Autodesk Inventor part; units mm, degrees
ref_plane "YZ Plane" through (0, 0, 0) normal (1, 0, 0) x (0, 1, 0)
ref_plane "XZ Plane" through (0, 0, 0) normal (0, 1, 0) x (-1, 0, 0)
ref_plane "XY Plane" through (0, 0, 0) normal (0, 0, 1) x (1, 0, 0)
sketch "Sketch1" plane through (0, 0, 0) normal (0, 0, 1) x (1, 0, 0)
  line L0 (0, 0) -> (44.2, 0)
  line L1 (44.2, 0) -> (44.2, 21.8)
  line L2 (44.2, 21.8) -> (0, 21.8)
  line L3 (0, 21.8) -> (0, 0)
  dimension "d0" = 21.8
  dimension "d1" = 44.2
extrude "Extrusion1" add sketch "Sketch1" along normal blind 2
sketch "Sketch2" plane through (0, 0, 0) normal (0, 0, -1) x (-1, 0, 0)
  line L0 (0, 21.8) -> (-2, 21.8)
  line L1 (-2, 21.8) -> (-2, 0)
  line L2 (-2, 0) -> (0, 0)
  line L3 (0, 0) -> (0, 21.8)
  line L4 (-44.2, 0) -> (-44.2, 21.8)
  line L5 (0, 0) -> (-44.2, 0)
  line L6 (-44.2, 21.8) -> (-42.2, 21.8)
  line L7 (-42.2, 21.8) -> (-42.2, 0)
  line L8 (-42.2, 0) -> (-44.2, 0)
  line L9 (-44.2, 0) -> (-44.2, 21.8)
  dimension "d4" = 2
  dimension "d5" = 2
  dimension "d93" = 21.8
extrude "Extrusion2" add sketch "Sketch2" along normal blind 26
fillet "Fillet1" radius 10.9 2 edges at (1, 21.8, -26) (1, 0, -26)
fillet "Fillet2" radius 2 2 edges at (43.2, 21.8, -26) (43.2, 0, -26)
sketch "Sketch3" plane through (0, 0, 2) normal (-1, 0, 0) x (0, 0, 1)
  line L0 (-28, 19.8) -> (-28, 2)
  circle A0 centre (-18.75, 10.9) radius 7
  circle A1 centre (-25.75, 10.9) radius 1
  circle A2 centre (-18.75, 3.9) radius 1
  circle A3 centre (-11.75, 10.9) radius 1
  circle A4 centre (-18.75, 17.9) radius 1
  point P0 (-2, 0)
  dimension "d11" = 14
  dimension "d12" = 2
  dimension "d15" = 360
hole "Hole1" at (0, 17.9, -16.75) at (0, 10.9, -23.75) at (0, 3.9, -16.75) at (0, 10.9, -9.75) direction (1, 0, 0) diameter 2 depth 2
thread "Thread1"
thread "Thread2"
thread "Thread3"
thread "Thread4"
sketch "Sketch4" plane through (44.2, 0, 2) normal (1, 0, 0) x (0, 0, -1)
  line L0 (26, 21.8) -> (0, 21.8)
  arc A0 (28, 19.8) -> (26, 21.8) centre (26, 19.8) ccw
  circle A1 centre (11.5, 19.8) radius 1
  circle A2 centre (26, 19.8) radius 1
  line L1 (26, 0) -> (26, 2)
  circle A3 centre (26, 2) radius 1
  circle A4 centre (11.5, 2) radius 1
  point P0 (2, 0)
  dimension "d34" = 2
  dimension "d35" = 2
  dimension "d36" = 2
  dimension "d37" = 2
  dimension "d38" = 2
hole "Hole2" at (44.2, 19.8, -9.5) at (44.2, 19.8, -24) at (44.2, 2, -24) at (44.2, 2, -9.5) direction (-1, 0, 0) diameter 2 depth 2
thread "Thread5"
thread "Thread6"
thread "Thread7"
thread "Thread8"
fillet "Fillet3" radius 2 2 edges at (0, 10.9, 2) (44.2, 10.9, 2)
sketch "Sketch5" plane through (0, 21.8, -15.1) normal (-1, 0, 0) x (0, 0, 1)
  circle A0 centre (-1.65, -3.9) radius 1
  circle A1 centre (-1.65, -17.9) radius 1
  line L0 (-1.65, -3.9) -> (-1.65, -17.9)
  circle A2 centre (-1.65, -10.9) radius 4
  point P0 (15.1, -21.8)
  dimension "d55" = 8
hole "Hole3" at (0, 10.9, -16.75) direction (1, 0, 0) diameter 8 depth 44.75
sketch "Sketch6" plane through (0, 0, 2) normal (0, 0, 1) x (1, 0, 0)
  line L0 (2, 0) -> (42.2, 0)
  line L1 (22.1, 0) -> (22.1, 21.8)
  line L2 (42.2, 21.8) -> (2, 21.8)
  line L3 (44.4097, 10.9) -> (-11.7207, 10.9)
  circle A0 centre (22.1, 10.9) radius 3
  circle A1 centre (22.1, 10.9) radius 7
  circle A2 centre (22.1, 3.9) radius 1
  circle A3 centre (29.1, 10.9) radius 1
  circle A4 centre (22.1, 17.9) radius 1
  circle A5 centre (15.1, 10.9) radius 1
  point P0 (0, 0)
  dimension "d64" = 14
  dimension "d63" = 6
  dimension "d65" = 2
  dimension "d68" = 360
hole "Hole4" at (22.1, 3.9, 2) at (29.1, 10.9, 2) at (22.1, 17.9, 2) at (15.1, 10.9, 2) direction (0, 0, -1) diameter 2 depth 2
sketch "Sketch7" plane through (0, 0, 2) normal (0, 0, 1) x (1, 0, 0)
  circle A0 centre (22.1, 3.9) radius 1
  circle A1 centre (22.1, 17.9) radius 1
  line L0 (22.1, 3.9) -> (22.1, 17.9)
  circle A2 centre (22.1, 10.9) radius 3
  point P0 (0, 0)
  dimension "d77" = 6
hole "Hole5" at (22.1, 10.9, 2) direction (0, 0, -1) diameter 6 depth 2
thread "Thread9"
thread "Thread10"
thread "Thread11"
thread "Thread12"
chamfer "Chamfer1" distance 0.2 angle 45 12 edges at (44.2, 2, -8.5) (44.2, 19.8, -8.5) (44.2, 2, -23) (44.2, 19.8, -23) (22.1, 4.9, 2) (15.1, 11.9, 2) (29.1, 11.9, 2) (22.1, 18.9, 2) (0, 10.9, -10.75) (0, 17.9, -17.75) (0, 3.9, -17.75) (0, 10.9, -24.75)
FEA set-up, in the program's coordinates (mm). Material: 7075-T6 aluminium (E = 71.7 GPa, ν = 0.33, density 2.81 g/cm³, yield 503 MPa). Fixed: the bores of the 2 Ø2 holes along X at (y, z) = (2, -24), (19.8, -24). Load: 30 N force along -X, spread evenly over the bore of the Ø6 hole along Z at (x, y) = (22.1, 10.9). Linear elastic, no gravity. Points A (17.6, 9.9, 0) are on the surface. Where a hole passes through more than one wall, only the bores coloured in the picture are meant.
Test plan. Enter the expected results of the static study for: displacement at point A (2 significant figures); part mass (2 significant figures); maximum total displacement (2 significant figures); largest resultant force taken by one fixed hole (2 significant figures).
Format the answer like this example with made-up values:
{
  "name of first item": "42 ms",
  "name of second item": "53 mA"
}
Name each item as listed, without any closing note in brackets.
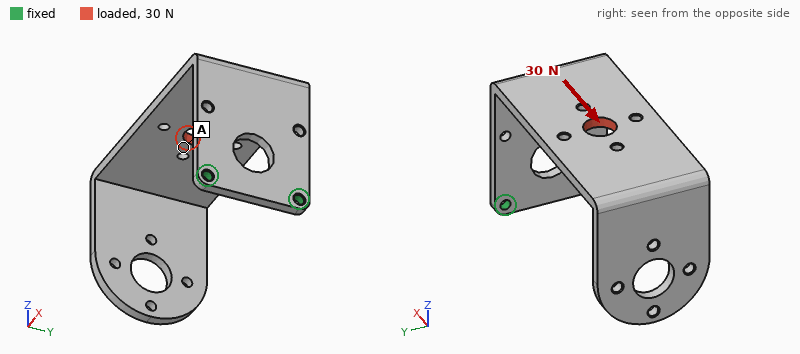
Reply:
{
  "displacement at point A": "0.38 mm",
  "part mass": "10 g",
  "maximum total displacement": "0.57 mm",
  "largest resultant force taken by one fixed hole": "15 N"
}
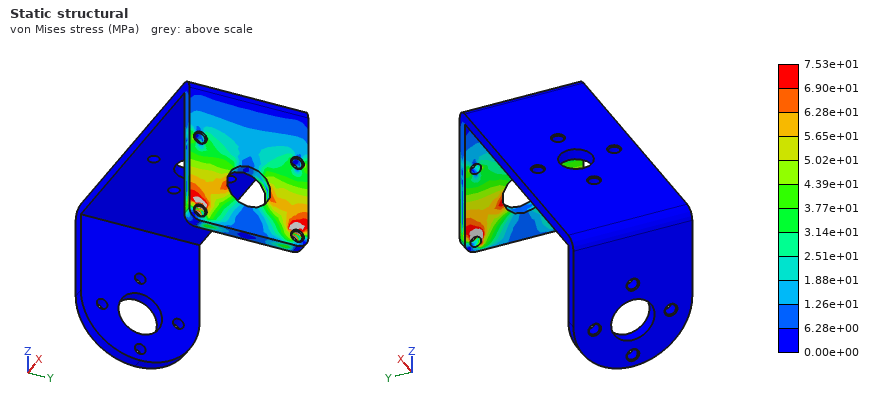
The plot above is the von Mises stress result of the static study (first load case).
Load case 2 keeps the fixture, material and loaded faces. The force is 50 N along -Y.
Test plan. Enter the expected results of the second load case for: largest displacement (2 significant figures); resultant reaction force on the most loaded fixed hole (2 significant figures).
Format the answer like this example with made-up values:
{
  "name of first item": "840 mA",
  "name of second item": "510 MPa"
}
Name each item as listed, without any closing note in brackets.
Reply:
{
  "largest displacement": "0.66 mm",
  "resultant reaction force on the most loaded fixed hole": "91 N"
}
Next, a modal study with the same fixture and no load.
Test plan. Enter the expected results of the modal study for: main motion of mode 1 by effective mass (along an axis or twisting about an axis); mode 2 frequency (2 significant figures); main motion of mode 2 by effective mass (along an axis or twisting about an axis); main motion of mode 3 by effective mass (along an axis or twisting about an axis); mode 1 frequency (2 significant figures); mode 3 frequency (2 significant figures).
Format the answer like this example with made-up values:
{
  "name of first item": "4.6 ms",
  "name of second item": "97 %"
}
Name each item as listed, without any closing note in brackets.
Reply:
{
  "main motion of mode 1 by effective mass": "along Z",
  "mode 2 frequency": "460 Hz",
  "main motion of mode 2 by effective mass": "along Y",
  "main motion of mode 3 by effective mass": "along X",
  "mode 1 frequency": "270 Hz",
  "mode 3 frequency": "830 Hz"
}
